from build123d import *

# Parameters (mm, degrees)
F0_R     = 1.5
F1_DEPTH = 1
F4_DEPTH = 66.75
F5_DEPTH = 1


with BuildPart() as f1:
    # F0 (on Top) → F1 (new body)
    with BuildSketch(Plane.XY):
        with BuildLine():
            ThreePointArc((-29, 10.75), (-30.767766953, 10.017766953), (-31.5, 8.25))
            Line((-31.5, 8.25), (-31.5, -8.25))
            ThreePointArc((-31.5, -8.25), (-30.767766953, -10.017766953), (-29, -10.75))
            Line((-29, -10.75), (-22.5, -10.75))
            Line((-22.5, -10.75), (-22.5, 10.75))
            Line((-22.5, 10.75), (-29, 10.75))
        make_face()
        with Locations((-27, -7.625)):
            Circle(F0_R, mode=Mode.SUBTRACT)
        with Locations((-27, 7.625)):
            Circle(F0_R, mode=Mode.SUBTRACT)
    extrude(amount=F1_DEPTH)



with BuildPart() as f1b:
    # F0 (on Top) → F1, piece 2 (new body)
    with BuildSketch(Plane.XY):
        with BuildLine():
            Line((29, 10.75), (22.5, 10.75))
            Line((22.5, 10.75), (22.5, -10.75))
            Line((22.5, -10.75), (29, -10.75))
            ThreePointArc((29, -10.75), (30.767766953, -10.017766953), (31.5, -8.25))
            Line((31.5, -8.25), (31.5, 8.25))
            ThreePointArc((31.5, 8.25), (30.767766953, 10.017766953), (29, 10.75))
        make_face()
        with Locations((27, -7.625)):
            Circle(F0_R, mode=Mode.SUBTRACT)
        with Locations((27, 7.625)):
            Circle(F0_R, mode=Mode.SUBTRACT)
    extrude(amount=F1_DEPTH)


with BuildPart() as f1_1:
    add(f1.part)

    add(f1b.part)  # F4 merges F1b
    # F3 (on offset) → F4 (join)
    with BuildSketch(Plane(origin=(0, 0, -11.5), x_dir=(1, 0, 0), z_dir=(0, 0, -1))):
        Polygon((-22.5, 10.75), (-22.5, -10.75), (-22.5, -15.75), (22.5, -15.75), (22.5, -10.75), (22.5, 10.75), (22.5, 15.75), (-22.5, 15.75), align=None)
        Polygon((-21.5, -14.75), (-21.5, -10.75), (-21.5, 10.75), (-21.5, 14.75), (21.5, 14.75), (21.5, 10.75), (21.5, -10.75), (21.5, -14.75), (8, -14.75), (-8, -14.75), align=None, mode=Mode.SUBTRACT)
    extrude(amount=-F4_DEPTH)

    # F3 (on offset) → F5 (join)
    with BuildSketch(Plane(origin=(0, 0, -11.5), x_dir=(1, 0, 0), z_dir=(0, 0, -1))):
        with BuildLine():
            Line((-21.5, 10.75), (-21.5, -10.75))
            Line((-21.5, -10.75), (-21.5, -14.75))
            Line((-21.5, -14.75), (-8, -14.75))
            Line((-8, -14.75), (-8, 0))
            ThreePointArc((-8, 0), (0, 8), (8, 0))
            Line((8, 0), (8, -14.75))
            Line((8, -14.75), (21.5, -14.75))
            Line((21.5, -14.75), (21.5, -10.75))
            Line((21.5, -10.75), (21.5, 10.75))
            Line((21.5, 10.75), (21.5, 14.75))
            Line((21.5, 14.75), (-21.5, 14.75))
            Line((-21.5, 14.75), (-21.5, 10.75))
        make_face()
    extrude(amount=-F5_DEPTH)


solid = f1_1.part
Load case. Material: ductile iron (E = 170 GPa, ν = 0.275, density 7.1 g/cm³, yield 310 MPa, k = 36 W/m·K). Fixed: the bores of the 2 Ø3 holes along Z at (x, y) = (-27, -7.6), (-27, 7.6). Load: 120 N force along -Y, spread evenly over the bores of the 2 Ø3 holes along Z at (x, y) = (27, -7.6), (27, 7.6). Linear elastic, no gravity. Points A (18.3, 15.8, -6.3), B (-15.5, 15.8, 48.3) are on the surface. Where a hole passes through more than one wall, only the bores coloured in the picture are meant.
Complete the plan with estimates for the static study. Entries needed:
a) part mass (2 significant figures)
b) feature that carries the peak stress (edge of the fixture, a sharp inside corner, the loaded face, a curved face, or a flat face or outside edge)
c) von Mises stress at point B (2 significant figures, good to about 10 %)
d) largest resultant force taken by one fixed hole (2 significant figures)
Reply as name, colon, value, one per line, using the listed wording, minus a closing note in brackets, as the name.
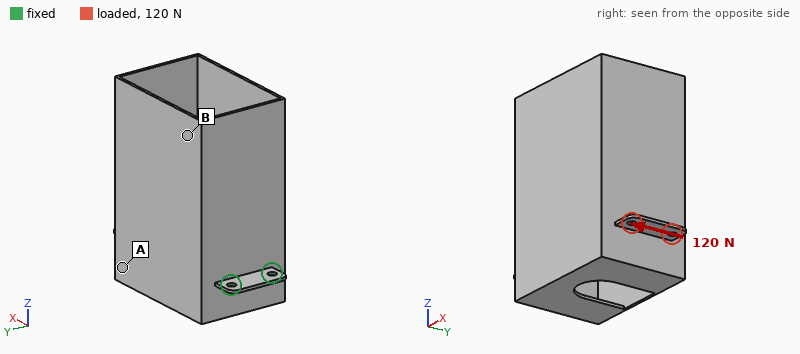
part mass: 80 g
feature that carries the peak stress: a flat face or outside edge
von Mises stress at point B: 31 MPa
largest resultant force taken by one fixed hole: 380 N
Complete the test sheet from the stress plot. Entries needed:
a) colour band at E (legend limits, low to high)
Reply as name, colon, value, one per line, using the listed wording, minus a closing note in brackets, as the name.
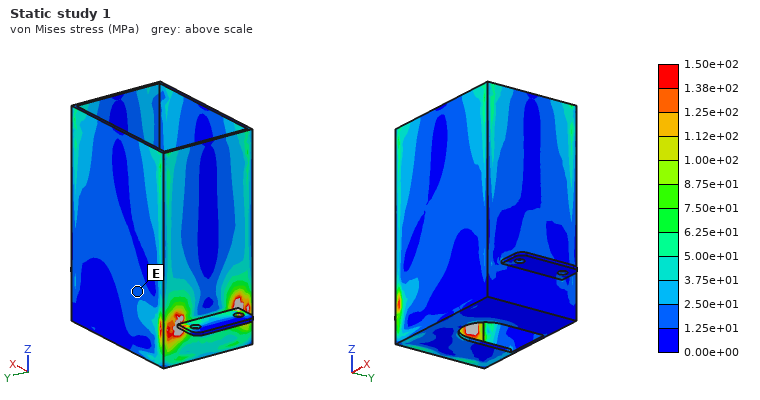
colour band at E: 1.25e+01 to 2.50e+01 MPa
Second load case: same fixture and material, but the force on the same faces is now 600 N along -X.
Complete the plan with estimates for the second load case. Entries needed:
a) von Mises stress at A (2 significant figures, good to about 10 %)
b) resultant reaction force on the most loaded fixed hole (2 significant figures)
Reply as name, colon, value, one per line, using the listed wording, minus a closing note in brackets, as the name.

von Mises stress at A: 46 MPa
resultant reaction force on the most loaded fixed hole: 350 N
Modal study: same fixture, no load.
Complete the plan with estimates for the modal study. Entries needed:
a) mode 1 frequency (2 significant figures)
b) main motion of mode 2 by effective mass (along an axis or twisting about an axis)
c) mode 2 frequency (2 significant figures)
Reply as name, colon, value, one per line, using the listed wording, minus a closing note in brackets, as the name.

mode 1 frequency: 110 Hz
main motion of mode 2 by effective mass: along Y
mode 2 frequency: 430 Hz
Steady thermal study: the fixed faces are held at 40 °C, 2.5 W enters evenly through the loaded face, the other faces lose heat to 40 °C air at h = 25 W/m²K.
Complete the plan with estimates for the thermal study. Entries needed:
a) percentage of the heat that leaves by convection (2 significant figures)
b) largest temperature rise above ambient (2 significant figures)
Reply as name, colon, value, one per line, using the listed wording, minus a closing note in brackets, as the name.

percentage of the heat that leaves by convection: 95 %
largest temperature rise above ambient: 42 K
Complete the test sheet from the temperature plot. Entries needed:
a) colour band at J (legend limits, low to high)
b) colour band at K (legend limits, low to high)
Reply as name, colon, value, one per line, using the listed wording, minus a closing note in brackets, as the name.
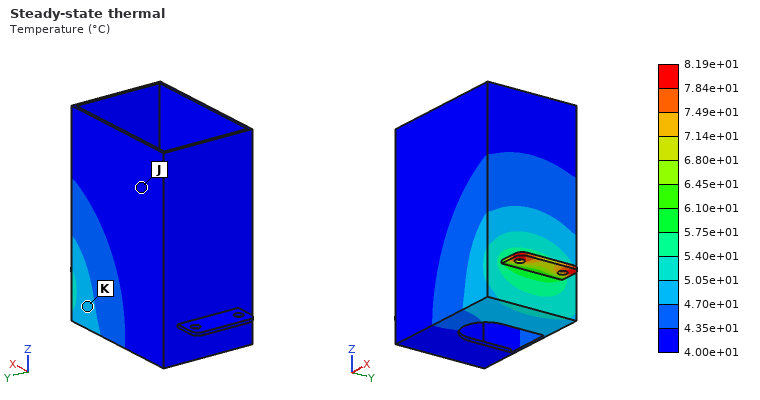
colour band at J: 4.00e+01 to 4.35e+01 °C
colour band at K: 4.70e+01 to 5.05e+01 °C
